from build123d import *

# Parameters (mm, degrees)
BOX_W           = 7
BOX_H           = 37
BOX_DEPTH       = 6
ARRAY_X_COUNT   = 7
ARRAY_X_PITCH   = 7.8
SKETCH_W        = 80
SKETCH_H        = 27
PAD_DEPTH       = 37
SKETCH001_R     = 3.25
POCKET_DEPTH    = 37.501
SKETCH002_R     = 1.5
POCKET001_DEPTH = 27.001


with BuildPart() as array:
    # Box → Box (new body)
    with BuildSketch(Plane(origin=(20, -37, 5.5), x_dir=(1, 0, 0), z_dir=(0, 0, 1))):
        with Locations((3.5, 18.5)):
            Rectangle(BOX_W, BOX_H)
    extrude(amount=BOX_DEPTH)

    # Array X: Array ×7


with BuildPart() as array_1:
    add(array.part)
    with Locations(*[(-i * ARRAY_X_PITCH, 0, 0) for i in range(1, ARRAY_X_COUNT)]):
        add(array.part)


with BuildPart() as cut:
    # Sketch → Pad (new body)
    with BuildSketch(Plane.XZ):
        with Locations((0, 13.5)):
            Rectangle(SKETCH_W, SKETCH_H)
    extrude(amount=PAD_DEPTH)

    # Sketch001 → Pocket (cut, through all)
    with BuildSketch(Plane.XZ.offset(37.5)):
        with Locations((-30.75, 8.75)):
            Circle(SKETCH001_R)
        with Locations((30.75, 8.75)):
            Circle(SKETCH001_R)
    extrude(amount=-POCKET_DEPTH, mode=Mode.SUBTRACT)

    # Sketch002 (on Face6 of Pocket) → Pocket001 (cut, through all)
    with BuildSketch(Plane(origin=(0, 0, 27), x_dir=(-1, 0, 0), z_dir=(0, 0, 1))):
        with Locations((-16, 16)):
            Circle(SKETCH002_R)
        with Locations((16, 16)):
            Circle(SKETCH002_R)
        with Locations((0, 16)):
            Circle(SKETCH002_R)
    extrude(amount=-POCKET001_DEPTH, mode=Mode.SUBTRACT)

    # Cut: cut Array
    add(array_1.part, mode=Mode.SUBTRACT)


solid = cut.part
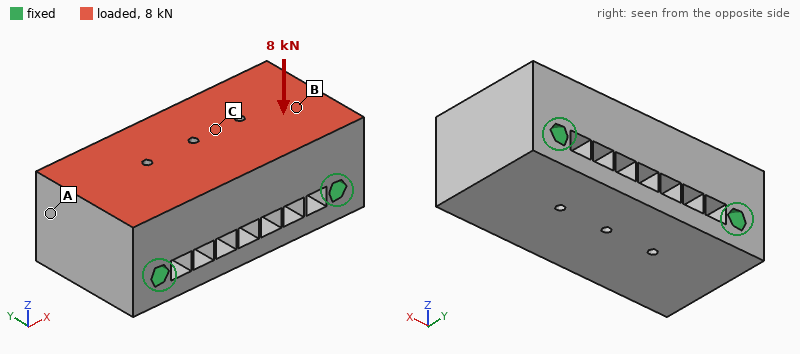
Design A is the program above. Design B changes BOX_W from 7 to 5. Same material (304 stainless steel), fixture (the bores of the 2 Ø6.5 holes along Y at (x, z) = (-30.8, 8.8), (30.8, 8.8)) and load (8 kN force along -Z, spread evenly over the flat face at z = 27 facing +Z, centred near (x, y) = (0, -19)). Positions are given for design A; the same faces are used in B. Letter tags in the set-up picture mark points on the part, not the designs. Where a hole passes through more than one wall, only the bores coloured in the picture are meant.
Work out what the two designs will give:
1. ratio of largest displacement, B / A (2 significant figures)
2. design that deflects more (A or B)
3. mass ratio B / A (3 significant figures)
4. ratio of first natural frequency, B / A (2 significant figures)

0.75
A
1.05
1.1
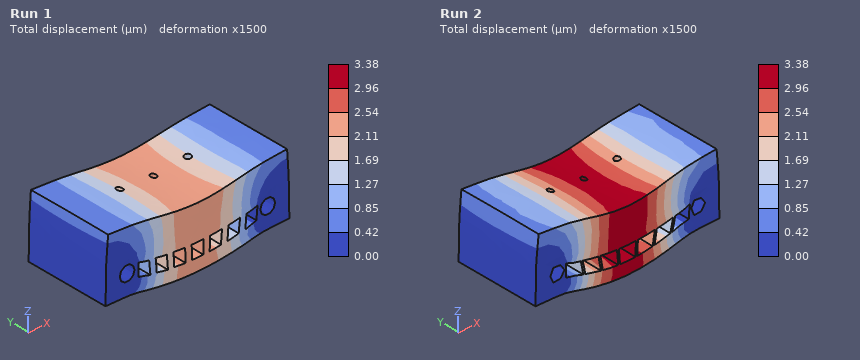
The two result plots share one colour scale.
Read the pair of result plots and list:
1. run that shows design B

Run 1
